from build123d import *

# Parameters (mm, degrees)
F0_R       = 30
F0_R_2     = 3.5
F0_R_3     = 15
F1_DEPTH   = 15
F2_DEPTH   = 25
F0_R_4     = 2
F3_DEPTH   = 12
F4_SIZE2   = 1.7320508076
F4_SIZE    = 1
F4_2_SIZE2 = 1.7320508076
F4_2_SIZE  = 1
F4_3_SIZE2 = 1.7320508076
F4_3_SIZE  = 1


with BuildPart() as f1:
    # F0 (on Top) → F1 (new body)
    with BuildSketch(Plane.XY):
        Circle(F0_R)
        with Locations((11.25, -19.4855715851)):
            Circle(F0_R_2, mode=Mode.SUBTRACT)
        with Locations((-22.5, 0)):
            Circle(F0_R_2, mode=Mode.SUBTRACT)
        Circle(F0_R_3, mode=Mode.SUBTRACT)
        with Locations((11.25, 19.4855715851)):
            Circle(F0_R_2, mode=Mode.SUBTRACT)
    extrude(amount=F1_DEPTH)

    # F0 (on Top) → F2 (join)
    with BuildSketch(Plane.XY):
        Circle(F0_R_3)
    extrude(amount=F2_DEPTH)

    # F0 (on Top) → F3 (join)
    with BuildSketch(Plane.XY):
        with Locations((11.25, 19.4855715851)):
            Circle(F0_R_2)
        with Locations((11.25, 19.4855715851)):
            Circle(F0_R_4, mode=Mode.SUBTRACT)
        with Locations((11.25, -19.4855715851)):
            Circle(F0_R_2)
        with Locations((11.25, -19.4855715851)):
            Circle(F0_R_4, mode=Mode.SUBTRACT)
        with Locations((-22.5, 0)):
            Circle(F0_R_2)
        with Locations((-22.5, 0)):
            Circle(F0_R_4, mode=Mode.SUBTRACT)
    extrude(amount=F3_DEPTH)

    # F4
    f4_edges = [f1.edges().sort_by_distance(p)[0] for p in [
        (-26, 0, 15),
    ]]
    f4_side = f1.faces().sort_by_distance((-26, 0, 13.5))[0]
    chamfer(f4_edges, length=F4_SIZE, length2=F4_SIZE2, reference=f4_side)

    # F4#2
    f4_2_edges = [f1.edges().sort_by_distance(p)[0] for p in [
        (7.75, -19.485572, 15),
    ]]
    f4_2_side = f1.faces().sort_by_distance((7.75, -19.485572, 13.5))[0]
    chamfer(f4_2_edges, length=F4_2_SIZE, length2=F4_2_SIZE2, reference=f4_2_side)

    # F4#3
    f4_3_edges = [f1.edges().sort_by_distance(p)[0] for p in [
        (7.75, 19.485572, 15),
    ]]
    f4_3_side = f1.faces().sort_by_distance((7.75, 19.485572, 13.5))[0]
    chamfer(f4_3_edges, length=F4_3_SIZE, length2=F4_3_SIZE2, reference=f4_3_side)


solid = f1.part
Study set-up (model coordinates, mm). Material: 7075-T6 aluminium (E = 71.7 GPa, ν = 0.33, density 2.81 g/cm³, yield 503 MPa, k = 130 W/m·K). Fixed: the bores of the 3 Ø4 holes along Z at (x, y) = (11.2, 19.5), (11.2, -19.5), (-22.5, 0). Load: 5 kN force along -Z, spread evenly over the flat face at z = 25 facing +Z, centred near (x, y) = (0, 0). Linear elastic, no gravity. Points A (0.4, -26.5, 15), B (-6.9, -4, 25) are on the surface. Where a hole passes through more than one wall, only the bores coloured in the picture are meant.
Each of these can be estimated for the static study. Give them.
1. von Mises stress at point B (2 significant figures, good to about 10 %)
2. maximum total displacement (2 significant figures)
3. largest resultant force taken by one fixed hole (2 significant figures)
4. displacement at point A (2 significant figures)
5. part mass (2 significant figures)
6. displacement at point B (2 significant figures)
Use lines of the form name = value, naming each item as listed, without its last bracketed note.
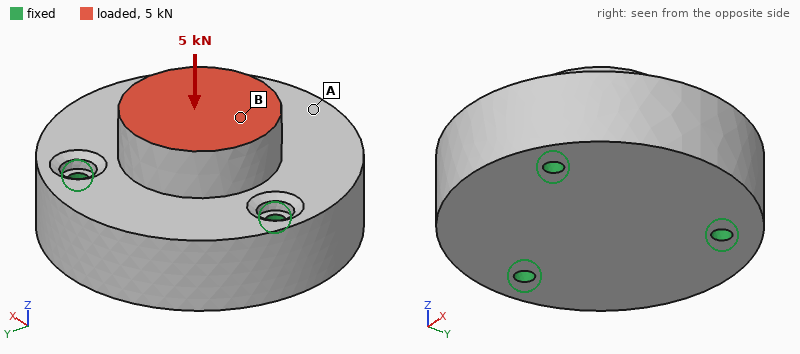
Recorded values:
von Mises stress at point B = 5.8 MPa
maximum total displacement = 4.8 µm
largest resultant force taken by one fixed hole = 1.7 kN
displacement at point A = 1.8 µm
part mass = 140 g
displacement at point B = 4.7 µm
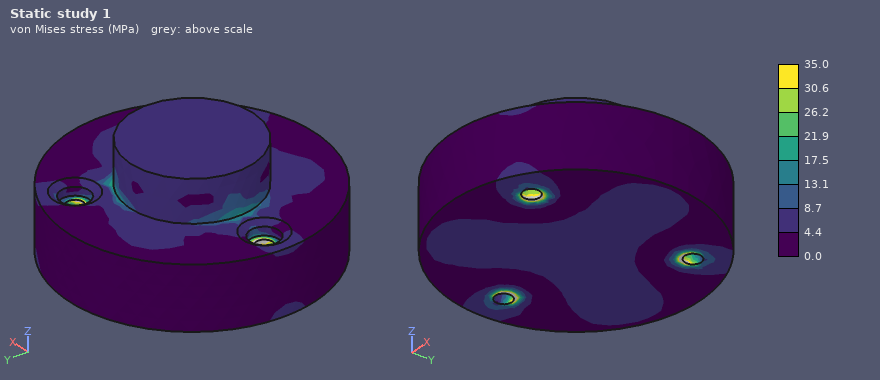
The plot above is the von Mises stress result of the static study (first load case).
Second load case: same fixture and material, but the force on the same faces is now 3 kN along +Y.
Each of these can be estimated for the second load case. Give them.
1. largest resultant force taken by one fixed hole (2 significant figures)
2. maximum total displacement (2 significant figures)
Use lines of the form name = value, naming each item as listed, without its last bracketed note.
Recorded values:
largest resultant force taken by one fixed hole = 1.7 kN
maximum total displacement = 7.7 µm
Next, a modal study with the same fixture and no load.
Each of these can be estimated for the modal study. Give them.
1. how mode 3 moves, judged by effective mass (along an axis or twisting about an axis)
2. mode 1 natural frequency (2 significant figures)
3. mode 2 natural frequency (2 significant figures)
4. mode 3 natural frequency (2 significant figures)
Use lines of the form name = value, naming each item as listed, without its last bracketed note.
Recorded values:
how mode 3 moves, judged by effective mass = along Z
mode 1 natural frequency = 18 kHz
mode 2 natural frequency = 18 kHz
mode 3 natural frequency = 19 kHz
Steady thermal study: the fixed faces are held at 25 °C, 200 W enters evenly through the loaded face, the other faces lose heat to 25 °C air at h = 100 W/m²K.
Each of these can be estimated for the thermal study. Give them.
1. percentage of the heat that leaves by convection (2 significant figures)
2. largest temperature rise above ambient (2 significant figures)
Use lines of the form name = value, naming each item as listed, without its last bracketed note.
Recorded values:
percentage of the heat that leaves by convection = 5.9 %
largest temperature rise above ambient = 49 K
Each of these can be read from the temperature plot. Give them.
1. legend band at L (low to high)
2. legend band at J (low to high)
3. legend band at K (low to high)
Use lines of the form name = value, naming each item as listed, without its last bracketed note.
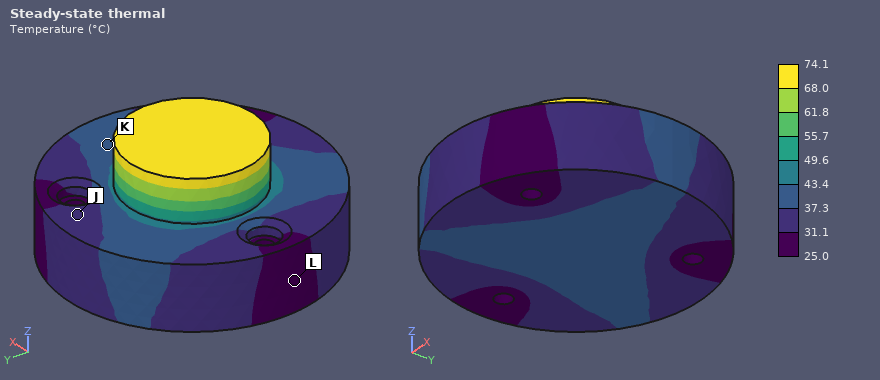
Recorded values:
legend band at L = 25.0 to 31.1 °C
legend band at J = 31.1 to 37.3 °C
legend band at K = 37.3 to 43.4 °C
